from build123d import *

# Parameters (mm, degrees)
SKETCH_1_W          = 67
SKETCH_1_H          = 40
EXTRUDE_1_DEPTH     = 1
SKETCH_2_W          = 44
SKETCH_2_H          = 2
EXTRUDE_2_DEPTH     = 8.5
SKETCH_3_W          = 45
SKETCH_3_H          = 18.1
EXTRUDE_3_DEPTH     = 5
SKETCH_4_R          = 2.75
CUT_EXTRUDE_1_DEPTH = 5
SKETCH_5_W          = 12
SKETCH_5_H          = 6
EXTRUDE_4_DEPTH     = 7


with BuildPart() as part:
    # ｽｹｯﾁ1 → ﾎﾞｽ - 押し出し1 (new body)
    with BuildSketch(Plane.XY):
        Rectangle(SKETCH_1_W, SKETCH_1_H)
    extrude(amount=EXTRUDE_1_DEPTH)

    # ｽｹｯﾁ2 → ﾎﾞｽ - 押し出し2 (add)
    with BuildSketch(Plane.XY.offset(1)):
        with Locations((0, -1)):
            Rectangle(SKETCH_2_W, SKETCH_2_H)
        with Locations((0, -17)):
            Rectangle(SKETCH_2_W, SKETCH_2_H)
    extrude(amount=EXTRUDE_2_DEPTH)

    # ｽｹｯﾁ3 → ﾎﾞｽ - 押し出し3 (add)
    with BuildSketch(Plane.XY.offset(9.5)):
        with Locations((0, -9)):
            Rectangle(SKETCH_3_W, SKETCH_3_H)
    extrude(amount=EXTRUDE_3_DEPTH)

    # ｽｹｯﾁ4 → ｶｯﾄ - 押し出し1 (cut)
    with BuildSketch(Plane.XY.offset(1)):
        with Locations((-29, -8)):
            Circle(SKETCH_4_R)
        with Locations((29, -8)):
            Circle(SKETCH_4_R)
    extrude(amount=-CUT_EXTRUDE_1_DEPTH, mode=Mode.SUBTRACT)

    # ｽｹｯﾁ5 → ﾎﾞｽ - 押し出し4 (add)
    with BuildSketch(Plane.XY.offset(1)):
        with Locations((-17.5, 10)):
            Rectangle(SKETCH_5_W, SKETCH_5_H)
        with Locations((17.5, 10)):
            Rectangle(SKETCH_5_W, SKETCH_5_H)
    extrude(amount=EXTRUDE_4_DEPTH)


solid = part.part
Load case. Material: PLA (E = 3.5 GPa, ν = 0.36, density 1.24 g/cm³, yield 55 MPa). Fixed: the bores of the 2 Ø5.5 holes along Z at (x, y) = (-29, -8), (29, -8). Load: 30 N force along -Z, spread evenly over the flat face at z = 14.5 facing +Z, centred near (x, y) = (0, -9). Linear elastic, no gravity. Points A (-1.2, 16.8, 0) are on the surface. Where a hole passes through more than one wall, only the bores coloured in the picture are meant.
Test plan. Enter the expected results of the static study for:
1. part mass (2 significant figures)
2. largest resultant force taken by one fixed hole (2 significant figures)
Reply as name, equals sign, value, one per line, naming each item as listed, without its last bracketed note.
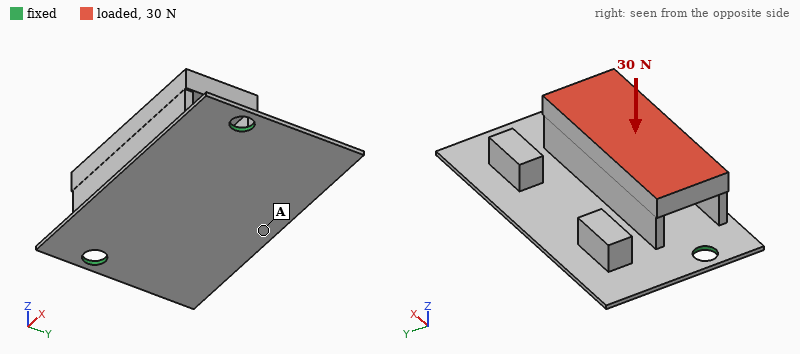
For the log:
part mass = 11 g
largest resultant force taken by one fixed hole = 17 N
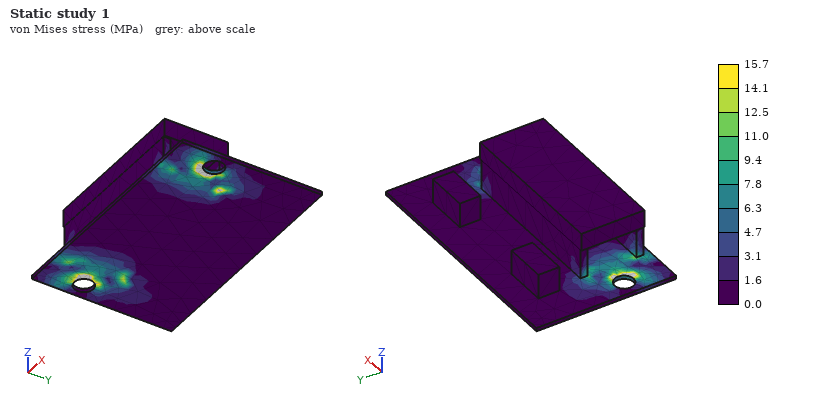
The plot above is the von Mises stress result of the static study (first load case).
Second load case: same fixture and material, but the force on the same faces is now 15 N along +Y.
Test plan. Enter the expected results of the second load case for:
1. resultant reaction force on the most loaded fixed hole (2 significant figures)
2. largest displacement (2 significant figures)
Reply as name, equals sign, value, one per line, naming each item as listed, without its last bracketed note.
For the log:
resultant reaction force on the most loaded fixed hole = 7.7 N
largest displacement = 0.88 mm
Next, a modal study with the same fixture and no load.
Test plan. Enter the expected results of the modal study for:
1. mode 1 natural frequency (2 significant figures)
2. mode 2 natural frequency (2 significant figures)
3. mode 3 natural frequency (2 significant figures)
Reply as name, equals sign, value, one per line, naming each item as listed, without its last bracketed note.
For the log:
mode 1 natural frequency = 270 Hz
mode 2 natural frequency = 600 Hz
mode 3 natural frequency = 610 Hz
